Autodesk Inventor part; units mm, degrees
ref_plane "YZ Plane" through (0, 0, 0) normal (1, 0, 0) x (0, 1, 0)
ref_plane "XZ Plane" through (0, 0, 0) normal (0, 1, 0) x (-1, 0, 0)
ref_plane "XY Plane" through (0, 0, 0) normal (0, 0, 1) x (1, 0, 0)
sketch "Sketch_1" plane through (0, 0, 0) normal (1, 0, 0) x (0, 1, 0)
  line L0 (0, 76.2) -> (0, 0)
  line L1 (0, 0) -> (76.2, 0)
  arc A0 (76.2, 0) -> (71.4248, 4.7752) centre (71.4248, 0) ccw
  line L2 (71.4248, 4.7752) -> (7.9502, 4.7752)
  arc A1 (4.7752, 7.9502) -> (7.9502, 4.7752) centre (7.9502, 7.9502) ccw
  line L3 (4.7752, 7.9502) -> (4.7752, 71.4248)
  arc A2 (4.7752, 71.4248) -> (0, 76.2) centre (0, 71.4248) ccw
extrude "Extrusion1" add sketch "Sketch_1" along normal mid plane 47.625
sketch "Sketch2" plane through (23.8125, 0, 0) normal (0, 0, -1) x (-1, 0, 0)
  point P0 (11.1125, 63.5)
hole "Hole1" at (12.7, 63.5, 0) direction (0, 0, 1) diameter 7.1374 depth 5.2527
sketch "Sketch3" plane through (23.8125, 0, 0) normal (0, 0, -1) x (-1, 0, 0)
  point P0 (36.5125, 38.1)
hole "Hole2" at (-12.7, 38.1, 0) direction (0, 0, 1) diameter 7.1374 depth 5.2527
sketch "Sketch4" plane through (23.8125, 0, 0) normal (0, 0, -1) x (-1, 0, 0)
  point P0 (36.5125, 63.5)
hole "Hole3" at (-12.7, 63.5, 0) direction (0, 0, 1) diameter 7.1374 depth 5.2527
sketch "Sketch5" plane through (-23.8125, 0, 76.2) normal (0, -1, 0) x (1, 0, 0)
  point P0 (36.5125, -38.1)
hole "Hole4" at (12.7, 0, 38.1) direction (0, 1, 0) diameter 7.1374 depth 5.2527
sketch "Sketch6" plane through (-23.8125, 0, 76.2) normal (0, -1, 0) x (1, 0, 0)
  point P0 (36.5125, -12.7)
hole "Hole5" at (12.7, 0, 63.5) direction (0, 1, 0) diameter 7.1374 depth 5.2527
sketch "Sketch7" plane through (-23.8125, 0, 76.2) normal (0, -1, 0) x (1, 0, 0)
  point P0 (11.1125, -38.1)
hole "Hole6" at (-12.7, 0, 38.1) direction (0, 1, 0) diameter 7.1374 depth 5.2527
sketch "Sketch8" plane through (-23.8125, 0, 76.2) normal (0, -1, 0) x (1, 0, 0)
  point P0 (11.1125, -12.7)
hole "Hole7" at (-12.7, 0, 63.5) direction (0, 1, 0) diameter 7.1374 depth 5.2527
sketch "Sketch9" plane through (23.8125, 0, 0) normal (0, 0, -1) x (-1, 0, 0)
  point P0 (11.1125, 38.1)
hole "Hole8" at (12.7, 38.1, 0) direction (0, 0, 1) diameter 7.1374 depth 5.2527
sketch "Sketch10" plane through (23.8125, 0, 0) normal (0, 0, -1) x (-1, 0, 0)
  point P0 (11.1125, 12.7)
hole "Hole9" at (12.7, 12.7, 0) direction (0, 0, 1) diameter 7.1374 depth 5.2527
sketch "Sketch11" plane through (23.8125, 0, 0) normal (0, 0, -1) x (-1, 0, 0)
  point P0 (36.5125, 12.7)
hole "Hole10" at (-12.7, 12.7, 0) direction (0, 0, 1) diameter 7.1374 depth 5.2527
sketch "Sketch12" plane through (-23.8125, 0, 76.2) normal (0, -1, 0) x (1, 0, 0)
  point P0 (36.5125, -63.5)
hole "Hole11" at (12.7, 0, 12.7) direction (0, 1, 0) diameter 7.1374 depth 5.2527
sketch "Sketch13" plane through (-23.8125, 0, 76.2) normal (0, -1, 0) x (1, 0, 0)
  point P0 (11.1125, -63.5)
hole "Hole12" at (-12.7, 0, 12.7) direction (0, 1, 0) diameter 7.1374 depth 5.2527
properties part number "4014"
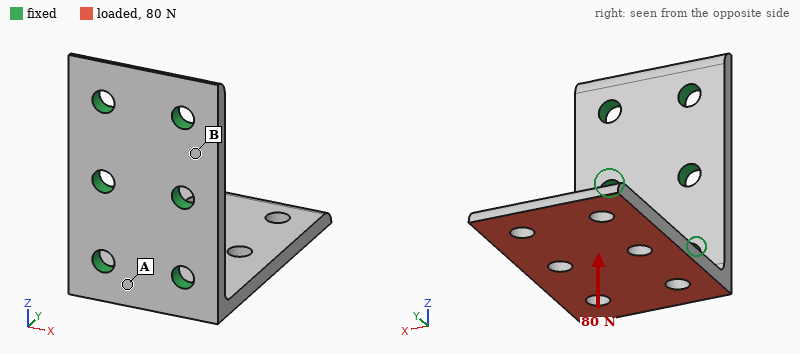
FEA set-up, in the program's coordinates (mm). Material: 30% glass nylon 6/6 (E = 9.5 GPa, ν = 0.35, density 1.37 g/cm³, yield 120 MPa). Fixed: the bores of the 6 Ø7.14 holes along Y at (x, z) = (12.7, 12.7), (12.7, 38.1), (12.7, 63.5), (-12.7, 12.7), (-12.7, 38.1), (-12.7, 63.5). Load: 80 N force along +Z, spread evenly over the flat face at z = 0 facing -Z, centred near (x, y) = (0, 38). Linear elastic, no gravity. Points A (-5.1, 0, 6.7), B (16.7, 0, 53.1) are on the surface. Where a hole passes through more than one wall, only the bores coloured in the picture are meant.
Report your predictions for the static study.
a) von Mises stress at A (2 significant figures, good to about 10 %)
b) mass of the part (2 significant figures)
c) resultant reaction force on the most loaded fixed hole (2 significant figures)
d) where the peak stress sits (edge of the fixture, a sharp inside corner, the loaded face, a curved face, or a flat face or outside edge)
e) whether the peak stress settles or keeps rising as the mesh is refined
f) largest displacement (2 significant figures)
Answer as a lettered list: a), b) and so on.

a) 9.5 MPa
b) 42 g
c) 40 N
d) edge of the fixture
e) keeps rising
f) 1.3 mm
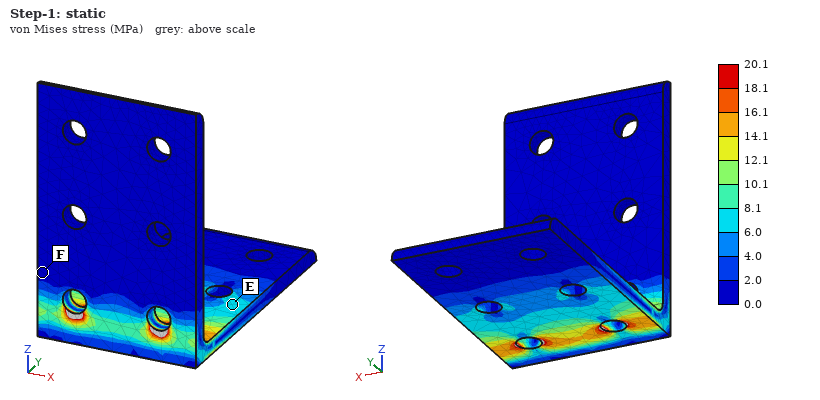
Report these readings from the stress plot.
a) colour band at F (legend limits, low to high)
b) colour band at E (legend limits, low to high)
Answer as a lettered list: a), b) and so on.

a) 0.0 to 2.0 MPa
b) 6.0 to 8.1 MPa
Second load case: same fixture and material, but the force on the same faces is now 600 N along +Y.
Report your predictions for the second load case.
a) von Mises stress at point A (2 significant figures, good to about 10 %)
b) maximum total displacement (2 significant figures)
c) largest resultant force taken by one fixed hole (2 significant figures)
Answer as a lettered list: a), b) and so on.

a) 13 MPa
b) 1.2 mm
c) 320 N
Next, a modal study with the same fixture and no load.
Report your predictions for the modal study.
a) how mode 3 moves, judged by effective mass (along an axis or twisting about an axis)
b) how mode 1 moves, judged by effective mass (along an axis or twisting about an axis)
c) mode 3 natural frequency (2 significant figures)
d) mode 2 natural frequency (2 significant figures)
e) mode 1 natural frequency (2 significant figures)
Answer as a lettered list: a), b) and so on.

a) along X
b) along Z
c) 1500 Hz
d) 1100 Hz
e) 340 Hz
